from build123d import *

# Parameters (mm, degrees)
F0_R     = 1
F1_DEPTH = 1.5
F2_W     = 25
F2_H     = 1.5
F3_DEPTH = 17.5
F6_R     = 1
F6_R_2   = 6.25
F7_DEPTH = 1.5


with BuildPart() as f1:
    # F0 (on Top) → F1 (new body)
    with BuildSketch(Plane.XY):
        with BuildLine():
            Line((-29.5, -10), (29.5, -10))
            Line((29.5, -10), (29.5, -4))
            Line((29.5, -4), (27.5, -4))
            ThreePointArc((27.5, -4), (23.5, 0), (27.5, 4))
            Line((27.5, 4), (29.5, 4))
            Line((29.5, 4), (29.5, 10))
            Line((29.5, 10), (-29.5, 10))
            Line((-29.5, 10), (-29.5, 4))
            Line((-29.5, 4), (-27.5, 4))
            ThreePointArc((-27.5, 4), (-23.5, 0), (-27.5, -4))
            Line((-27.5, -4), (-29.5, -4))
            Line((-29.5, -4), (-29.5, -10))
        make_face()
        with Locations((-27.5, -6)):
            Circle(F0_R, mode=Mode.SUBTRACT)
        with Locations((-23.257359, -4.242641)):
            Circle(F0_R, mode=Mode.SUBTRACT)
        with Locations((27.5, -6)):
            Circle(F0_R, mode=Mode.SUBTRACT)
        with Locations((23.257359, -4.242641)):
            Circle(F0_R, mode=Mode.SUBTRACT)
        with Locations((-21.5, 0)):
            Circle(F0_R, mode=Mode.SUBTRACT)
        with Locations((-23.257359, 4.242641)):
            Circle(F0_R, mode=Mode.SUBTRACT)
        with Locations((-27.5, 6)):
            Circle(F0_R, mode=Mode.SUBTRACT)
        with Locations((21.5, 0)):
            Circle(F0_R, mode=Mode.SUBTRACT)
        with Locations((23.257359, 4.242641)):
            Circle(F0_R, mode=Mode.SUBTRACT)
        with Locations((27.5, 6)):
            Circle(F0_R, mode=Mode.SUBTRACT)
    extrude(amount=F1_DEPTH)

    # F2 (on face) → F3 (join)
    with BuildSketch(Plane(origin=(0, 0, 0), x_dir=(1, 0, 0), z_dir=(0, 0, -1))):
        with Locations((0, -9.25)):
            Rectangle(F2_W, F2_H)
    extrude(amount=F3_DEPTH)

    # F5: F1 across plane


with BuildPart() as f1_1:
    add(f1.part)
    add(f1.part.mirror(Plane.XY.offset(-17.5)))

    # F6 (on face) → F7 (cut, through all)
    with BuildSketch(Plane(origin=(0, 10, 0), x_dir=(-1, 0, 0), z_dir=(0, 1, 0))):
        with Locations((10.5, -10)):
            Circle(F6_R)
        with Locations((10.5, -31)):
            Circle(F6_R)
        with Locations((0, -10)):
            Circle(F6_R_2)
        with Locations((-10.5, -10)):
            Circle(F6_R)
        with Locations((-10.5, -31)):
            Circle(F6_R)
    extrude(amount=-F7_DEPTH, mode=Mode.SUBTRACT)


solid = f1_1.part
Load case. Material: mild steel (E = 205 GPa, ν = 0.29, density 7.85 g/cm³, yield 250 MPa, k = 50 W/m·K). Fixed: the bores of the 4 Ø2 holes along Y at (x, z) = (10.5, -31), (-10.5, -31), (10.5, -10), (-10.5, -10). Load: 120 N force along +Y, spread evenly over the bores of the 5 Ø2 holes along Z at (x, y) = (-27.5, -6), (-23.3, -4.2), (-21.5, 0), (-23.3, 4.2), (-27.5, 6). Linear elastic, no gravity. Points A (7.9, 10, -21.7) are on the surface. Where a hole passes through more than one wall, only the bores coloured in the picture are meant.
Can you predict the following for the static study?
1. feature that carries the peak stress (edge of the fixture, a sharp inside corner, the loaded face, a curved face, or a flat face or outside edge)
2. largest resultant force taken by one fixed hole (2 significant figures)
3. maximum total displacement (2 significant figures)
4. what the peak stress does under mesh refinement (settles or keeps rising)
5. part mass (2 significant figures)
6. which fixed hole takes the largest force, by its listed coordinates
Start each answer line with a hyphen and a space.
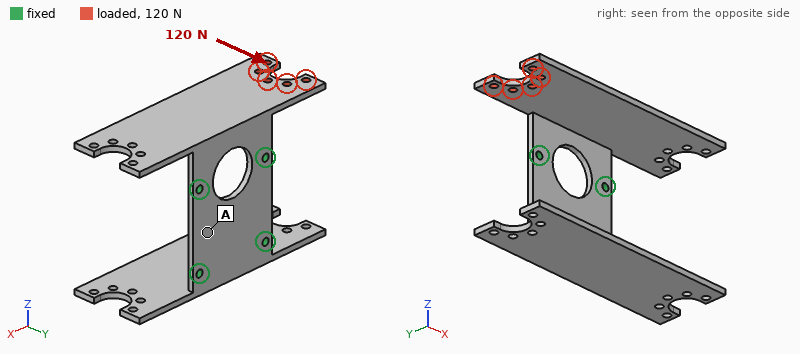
- edge of the fixture
- 200 N
- 0.32 mm
- keeps rising
- 34 g
- (-10.5, -10)
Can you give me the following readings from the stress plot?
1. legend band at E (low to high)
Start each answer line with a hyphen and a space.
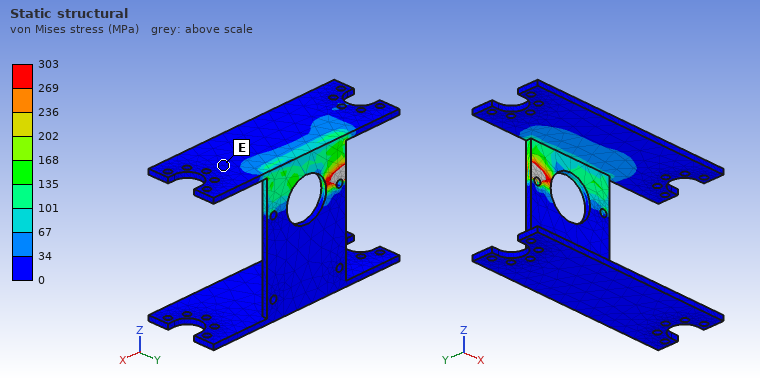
- 0 to 34 MPa
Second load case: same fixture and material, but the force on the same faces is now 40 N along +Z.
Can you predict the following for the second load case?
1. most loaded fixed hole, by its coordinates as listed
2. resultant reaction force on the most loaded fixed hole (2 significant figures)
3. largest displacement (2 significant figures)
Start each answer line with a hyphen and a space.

- (-10.5, -10)
- 66 N
- 0.23 mm
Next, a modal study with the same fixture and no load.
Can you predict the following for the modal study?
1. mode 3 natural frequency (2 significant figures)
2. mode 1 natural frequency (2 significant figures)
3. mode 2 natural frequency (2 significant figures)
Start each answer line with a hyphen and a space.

- 1600 Hz
- 1000 Hz
- 1600 Hz
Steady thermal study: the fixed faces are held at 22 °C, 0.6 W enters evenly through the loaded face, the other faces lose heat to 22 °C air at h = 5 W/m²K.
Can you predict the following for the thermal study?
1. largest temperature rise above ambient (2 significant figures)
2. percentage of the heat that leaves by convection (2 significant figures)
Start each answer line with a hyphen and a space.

- 14 K
- 15 %
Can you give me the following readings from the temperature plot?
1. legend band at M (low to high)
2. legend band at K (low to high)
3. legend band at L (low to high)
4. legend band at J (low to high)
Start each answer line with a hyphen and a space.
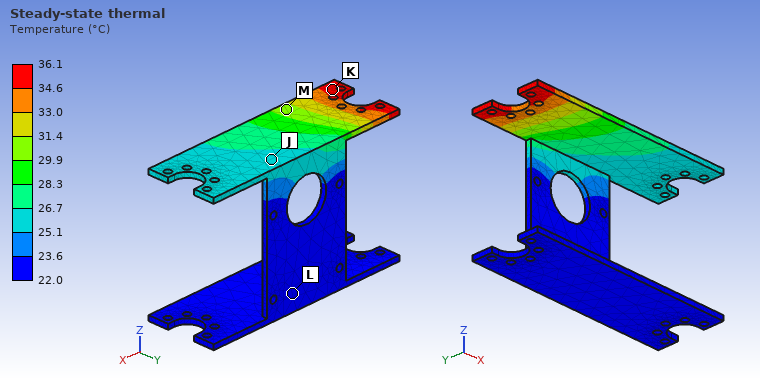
- 29.9 to 31.4 °C
- 34.6 to 36.1 °C
- 22.0 to 23.6 °C
- 25.1 to 26.7 °C
